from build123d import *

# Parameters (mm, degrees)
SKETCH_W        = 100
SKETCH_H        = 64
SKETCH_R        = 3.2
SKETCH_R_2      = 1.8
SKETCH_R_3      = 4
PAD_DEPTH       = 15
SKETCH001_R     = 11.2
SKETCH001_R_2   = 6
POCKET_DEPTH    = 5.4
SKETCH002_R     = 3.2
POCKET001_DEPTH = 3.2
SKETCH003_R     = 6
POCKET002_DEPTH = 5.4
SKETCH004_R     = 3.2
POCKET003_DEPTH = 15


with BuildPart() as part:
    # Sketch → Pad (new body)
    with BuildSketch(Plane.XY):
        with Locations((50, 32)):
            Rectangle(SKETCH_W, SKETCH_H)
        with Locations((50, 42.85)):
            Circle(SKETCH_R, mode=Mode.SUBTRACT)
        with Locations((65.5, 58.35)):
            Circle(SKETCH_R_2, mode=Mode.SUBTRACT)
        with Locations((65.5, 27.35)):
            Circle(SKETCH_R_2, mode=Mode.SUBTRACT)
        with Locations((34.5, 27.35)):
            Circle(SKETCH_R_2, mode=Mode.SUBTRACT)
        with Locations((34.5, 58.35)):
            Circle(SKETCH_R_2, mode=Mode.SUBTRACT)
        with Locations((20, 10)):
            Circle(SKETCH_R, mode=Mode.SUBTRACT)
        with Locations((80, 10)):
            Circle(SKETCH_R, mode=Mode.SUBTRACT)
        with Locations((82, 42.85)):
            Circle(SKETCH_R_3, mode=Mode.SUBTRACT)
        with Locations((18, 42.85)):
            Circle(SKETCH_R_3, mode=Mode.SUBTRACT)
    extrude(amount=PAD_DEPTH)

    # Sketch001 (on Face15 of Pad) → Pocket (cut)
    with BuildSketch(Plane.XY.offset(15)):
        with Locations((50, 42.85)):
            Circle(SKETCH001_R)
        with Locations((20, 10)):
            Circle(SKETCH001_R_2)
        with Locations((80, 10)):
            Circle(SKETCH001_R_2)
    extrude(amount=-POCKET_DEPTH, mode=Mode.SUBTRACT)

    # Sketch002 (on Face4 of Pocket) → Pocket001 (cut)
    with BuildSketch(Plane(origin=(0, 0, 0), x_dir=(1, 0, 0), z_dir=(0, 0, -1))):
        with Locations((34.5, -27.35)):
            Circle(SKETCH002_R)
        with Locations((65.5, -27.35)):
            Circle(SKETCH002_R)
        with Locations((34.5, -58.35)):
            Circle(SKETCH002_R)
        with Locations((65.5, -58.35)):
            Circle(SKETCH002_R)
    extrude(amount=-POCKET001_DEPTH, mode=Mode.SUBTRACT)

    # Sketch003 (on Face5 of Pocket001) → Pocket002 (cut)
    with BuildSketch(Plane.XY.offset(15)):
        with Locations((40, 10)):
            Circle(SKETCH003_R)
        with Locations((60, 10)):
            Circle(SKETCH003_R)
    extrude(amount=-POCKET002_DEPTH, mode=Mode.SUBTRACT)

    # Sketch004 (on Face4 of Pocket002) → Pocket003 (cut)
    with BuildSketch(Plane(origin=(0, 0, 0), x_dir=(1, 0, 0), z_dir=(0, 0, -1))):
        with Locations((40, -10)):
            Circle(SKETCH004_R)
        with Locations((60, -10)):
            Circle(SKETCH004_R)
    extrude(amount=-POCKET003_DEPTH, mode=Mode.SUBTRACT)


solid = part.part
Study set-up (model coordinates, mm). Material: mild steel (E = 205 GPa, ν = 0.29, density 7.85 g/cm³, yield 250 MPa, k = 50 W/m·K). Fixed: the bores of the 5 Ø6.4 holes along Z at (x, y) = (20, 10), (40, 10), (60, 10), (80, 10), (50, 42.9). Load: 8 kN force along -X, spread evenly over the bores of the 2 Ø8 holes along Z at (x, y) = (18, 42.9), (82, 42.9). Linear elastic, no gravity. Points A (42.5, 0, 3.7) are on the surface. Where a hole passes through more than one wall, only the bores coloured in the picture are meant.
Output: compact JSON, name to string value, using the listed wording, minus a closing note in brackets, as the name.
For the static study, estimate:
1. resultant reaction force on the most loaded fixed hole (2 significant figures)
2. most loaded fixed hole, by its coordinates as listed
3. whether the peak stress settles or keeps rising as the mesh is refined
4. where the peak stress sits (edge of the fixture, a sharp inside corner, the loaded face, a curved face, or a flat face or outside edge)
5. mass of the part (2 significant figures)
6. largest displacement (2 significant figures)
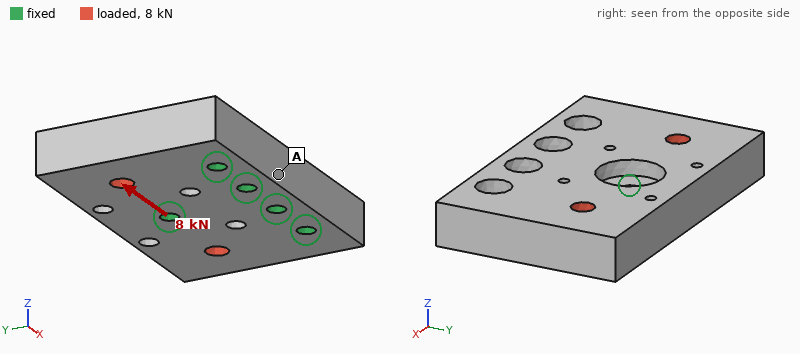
{"resultant reaction force on the most loaded fixed hole": "5.4 kN", "most loaded fixed hole, by its coordinates as listed": "(50, 42.9)", "whether the peak stress settles or keeps rising as the mesh is refined": "keeps rising", "where the peak stress sits": "edge of the fixture", "mass of the part": "690 g", "largest displacement": "3.3 µm"}
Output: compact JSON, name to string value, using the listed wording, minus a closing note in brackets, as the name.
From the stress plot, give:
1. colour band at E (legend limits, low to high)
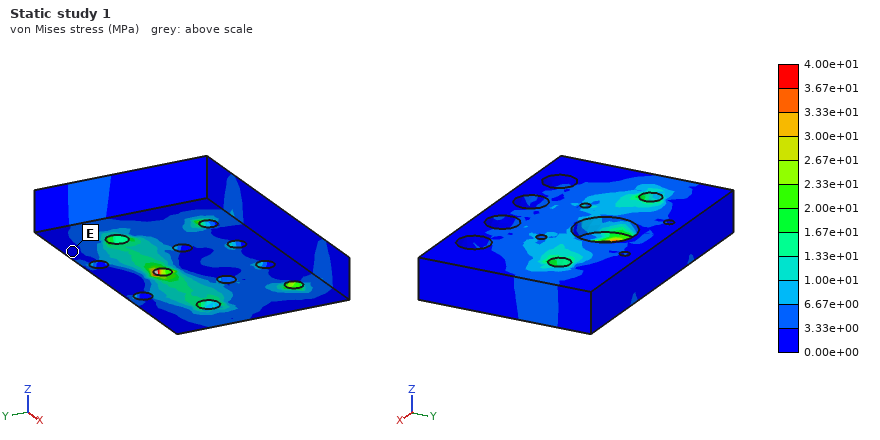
{"colour band at E": "0.00e+00 to 3.33e+00 MPa"}
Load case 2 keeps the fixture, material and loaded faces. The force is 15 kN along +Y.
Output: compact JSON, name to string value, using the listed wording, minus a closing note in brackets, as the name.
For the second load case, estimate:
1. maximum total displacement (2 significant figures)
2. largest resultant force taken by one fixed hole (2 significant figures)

{"maximum total displacement": "4.1 µm", "largest resultant force taken by one fixed hole": "4.5 kN"}
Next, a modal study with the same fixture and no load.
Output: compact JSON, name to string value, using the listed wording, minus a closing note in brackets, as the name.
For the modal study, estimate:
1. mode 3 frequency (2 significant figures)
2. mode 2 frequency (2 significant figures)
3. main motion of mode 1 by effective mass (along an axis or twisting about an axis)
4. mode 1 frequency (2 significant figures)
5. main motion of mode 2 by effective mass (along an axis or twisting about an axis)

{"mode 3 frequency": "13 kHz", "mode 2 frequency": "5800 Hz", "main motion of mode 1 by effective mass": "twisting about Y", "mode 1 frequency": "5200 Hz", "main motion of mode 2 by effective mass": "along Z"}
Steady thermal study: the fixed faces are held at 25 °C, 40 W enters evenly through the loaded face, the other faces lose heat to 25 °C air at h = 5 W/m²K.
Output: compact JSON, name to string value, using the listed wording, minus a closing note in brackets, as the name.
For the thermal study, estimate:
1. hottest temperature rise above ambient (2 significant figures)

{"hottest temperature rise above ambient": "20 K"}
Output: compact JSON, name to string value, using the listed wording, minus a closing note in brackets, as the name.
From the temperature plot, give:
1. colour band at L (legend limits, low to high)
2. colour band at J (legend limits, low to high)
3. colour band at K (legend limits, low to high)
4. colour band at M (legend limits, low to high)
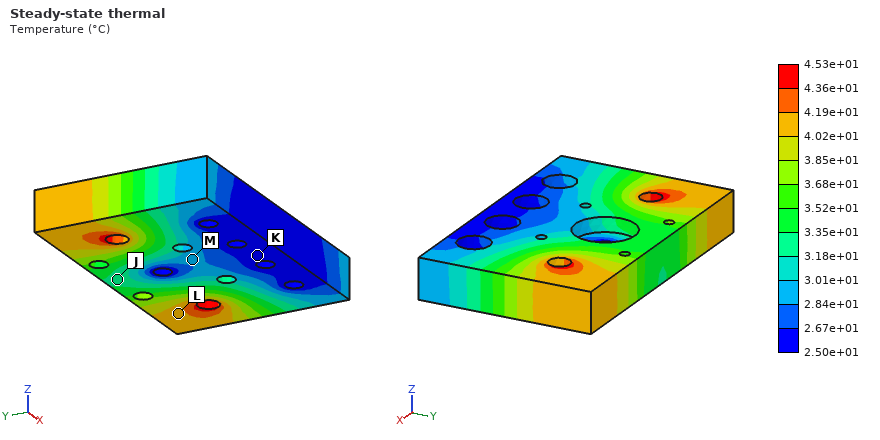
{"colour band at L": "4.02e+01 to 4.19e+01 °C", "colour band at J": "3.18e+01 to 3.35e+01 °C", "colour band at K": "2.50e+01 to 2.67e+01 °C", "colour band at M": "2.84e+01 to 3.01e+01 °C"}
